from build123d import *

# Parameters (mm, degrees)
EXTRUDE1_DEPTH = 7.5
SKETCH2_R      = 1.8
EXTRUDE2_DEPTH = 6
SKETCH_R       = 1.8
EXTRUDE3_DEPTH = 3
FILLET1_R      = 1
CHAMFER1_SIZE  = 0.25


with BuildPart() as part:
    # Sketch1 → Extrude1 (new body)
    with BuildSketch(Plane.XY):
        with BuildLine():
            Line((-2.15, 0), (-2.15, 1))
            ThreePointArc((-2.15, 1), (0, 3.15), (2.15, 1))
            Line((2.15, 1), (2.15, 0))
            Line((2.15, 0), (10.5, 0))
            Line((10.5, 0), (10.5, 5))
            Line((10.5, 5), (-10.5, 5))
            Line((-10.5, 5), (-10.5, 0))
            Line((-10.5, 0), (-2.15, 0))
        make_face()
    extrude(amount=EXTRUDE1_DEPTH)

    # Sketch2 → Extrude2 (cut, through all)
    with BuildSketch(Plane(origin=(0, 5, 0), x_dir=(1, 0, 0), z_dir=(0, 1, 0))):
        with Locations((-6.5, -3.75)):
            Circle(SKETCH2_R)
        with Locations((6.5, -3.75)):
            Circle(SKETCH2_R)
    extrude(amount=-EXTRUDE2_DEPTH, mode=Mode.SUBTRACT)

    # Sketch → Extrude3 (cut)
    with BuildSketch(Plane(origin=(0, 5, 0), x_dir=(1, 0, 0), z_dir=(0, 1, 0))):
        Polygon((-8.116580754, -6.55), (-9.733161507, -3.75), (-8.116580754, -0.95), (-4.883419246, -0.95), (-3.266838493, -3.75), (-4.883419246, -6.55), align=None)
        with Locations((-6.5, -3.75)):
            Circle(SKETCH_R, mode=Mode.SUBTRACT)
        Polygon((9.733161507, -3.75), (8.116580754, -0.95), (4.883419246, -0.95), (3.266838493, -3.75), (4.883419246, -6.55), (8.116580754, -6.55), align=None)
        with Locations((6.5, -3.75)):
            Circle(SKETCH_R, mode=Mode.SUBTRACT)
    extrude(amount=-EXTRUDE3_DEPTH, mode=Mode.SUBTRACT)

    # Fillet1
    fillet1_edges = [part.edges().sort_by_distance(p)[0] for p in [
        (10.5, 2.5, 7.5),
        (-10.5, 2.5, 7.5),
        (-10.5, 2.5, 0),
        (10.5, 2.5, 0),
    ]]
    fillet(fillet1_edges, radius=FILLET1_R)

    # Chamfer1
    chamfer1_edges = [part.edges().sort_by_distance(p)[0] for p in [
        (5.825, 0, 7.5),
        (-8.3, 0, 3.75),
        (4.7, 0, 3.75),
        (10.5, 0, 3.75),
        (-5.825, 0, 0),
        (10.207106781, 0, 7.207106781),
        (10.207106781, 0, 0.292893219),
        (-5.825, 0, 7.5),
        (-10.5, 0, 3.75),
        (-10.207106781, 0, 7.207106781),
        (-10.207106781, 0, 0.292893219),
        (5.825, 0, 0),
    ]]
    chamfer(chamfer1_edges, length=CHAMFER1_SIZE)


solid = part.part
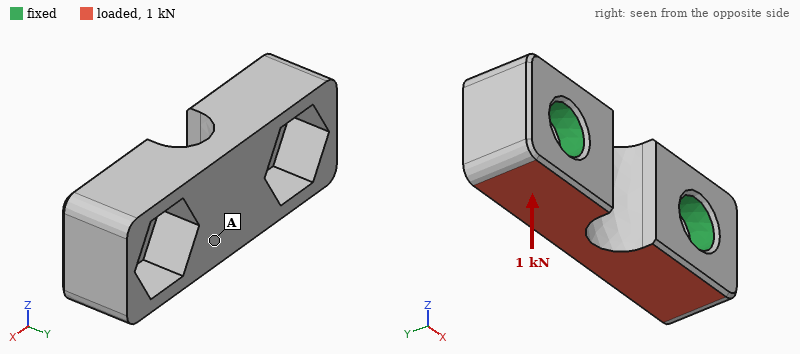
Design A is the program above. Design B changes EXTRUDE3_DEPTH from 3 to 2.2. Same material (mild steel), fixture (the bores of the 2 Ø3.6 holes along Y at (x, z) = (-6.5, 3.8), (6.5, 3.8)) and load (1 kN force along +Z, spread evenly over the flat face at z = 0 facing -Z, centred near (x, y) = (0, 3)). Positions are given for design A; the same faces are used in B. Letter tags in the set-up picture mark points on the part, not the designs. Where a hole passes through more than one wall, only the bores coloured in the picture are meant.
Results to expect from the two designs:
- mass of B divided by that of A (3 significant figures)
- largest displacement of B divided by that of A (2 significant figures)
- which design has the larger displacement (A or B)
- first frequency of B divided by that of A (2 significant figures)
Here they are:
1.06
0.58
A
1.3
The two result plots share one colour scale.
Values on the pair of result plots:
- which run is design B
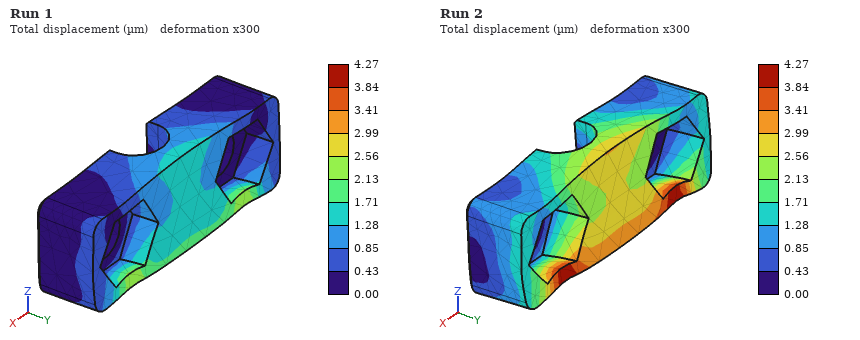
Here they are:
Run 1
